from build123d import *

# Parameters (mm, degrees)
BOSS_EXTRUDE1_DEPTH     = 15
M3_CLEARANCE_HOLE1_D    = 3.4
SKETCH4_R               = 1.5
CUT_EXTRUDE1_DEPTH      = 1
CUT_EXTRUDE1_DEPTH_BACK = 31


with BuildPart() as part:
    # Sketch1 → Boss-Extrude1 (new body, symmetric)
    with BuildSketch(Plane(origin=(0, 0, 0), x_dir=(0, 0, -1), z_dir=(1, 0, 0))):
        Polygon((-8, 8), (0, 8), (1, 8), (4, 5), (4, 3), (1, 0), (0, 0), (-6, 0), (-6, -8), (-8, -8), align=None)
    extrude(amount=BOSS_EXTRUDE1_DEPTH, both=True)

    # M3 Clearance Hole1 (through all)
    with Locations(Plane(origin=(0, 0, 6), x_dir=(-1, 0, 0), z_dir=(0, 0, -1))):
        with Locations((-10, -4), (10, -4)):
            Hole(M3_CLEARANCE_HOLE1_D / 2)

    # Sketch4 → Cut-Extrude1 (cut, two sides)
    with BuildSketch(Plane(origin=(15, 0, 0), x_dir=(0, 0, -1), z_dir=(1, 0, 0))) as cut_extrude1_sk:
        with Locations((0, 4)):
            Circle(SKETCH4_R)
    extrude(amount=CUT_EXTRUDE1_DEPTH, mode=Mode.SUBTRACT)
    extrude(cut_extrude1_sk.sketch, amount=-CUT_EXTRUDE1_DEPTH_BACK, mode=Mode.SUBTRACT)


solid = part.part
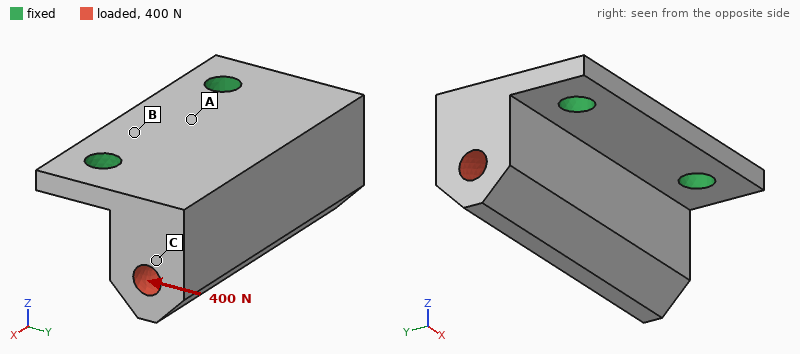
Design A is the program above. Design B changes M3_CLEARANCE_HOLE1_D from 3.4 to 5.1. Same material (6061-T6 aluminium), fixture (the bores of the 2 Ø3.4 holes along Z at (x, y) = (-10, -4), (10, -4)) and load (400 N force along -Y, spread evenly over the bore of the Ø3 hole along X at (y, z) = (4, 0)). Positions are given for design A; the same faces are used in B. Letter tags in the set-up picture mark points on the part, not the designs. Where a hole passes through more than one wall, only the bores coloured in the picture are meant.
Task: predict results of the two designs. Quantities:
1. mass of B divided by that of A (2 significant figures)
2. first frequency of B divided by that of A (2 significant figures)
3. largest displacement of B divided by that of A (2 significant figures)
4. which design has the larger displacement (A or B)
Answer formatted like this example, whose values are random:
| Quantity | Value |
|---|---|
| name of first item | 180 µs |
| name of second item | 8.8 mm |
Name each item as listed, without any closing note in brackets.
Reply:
| Quantity | Value |
|---|---|
| mass of B divided by that of A | 0.98 |
| first frequency of B divided by that of A | 1.2 |
| largest displacement of B divided by that of A | 0.73 |
| which design has the larger displacement | A |
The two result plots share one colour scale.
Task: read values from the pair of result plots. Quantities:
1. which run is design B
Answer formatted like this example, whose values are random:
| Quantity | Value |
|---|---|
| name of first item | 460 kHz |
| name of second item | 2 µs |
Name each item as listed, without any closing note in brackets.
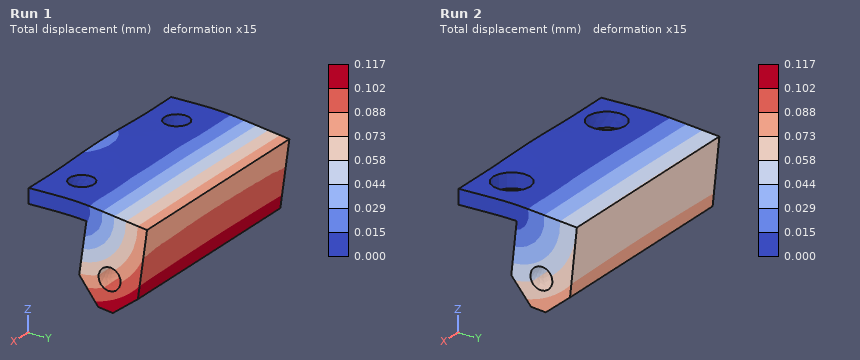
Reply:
| Quantity | Value |
|---|---|
| which run is design B | Run 2 |
